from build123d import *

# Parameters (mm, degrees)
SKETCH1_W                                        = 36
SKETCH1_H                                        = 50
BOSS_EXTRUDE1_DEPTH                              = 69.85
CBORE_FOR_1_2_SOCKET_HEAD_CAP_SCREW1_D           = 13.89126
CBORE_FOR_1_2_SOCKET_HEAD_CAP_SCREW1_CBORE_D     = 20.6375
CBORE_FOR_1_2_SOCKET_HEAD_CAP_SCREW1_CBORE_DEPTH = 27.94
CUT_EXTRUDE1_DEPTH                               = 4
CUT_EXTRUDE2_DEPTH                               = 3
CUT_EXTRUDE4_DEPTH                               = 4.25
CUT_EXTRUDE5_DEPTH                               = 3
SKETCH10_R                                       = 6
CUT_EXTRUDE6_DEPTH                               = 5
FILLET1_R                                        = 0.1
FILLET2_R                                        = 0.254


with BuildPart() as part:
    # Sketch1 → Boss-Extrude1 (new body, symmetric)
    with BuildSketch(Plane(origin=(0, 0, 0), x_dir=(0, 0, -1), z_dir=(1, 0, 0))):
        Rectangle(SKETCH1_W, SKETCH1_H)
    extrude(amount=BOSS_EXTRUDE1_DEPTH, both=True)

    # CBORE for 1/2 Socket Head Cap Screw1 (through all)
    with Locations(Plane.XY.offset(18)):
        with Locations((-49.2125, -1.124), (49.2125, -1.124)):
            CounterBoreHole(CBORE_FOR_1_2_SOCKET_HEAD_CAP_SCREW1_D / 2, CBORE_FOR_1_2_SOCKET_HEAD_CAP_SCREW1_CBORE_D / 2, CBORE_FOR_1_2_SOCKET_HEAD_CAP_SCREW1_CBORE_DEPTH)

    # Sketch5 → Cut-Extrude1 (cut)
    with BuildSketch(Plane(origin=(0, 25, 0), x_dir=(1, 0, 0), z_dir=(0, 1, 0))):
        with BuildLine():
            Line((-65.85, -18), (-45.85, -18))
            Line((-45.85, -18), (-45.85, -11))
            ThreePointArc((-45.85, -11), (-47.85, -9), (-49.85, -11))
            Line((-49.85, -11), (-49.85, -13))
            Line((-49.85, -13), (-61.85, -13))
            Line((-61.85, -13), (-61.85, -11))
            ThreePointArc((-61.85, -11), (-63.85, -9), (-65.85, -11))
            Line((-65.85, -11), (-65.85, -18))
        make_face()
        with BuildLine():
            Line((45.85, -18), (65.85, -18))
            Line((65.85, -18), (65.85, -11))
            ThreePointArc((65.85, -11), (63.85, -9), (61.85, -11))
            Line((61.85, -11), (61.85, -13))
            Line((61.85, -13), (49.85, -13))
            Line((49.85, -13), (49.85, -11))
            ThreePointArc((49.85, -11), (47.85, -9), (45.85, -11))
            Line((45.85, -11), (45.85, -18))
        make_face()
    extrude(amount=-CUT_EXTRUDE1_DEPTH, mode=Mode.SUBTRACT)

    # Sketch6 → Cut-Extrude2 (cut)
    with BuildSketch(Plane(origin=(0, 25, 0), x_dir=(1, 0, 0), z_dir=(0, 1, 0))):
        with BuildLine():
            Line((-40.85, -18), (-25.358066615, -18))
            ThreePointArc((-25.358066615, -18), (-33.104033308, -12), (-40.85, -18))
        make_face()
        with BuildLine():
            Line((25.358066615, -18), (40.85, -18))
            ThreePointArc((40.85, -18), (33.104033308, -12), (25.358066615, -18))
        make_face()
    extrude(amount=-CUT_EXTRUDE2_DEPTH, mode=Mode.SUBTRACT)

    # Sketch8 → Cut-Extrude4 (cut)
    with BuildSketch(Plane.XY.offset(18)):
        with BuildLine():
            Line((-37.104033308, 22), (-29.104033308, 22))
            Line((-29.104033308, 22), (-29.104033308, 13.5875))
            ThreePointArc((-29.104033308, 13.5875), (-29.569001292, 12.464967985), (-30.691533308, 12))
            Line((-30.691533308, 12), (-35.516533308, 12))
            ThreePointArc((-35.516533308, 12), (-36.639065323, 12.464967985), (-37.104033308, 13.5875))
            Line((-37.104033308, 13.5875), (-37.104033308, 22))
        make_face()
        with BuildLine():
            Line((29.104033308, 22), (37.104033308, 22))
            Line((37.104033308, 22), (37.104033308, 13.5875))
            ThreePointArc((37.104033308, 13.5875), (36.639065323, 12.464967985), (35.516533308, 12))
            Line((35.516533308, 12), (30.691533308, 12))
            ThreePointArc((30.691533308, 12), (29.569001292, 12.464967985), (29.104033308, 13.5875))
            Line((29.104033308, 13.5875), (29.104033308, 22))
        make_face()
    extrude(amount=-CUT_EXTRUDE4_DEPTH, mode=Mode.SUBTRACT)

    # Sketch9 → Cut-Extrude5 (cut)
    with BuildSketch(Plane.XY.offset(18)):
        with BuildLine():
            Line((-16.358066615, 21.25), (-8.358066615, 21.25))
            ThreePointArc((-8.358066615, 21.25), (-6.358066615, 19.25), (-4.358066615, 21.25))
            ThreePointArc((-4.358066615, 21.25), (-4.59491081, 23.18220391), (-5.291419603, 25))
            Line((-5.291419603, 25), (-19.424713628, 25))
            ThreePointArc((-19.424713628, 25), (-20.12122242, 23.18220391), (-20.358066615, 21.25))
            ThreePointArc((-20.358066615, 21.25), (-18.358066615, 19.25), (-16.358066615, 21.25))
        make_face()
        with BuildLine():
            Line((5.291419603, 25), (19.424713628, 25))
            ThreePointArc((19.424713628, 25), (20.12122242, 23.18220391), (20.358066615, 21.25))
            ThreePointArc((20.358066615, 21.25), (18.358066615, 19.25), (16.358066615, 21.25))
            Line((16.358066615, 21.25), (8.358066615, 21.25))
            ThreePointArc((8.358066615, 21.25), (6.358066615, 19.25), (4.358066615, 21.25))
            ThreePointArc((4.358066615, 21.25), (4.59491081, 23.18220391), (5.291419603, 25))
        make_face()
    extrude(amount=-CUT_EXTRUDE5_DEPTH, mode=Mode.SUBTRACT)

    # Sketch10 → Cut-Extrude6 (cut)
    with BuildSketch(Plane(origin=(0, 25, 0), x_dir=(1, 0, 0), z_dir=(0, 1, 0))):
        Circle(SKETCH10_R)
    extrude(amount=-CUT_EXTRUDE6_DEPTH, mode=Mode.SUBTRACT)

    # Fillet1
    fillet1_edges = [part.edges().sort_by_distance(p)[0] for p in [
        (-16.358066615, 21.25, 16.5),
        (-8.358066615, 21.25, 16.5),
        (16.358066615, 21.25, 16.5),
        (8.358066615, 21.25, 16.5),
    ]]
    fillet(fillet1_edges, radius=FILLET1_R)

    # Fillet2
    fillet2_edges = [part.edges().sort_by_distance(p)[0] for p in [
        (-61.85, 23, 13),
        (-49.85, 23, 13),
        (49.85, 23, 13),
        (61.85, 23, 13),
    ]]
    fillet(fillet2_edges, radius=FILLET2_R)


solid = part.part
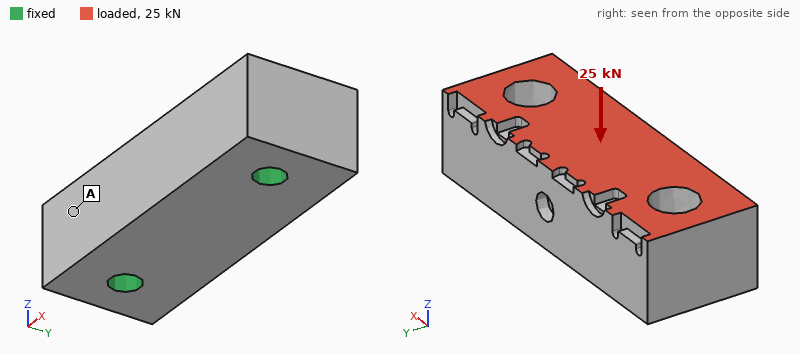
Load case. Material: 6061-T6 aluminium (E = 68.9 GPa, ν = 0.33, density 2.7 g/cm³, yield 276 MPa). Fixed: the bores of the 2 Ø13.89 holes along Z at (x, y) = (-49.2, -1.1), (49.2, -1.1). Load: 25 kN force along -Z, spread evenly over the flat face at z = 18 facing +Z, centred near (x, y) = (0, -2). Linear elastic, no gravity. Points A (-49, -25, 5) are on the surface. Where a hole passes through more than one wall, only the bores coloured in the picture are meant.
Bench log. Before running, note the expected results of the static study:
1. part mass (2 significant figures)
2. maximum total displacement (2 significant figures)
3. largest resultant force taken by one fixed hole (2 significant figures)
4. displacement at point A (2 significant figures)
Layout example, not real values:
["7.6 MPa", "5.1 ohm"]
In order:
["610 g", "26 µm", "13 kN", "14 µm"]
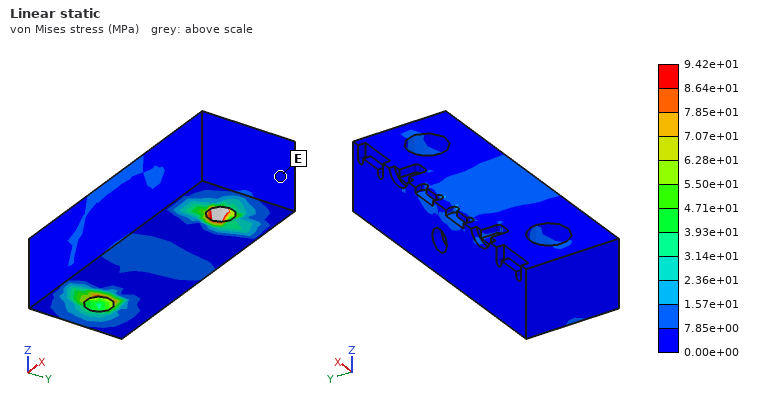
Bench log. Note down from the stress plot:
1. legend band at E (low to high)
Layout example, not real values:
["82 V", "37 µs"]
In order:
["0.00e+00 to 7.85e+00 MPa"]
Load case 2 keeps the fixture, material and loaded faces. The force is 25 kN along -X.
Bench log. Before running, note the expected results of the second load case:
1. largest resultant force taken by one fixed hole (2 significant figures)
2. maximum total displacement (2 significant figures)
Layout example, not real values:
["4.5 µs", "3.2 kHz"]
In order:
["15 kN", "30 µm"]
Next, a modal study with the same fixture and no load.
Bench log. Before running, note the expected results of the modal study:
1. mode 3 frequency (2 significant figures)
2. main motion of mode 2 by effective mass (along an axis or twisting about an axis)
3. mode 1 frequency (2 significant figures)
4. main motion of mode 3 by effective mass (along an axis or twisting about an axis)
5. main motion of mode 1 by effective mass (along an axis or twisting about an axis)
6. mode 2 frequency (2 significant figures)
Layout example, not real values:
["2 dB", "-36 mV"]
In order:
["8200 Hz", "along Z", "3400 Hz", "twisting about Z", "along Y", "7600 Hz"]
